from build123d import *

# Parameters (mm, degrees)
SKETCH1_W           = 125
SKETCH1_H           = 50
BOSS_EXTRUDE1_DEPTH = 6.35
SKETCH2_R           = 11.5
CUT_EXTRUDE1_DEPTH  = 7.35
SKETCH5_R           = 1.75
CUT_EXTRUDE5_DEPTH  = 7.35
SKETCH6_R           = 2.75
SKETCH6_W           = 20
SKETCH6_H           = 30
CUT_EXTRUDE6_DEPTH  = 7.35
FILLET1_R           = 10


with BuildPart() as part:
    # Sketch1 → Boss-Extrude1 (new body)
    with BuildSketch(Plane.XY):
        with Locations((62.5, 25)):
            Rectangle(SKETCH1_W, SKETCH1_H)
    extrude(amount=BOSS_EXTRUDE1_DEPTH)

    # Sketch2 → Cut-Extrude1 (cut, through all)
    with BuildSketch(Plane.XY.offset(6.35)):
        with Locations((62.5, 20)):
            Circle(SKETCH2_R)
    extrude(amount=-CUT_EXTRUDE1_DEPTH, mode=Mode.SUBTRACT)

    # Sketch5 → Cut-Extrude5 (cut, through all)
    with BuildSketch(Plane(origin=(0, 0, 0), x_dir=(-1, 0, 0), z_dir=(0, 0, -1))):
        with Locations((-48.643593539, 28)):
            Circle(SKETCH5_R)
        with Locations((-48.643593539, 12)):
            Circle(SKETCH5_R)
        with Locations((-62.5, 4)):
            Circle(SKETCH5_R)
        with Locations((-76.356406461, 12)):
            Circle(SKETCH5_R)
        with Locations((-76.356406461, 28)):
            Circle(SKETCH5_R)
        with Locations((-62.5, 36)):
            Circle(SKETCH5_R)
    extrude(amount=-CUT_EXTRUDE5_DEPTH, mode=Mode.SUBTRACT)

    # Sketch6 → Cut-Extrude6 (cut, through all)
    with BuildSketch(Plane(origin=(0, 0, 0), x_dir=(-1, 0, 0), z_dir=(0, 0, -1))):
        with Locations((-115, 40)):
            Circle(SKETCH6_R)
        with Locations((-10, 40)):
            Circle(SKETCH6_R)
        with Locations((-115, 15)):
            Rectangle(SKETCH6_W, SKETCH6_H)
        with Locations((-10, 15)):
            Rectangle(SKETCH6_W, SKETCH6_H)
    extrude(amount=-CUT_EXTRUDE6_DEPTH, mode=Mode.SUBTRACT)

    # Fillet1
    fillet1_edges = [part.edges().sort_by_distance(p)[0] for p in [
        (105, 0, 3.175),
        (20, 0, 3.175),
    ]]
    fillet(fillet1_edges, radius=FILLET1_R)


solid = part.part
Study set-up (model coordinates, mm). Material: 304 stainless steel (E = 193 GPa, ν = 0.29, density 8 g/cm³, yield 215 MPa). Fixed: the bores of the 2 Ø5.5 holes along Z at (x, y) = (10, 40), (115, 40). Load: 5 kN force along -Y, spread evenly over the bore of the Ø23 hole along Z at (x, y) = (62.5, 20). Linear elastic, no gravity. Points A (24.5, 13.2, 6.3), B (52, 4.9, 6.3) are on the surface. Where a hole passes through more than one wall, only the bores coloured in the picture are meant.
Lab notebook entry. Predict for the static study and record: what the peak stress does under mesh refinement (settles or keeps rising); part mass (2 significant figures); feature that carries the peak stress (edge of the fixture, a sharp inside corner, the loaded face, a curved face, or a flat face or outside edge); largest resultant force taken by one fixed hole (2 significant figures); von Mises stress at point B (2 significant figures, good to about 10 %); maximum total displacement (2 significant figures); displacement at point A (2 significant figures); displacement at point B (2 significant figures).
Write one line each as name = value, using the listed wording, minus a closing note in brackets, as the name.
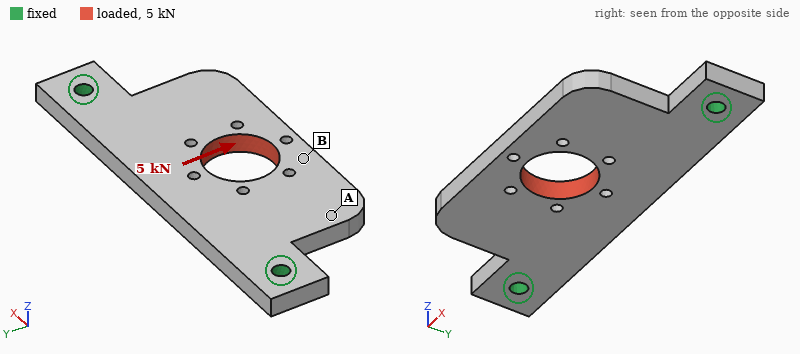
what the peak stress does under mesh refinement = keeps rising
part mass = 230 g
feature that carries the peak stress = edge of the fixture
largest resultant force taken by one fixed hole = 2.9 kN
von Mises stress at point B = 34 MPa
maximum total displacement = 19 µm
displacement at point A = 11 µm
displacement at point B = 16 µm
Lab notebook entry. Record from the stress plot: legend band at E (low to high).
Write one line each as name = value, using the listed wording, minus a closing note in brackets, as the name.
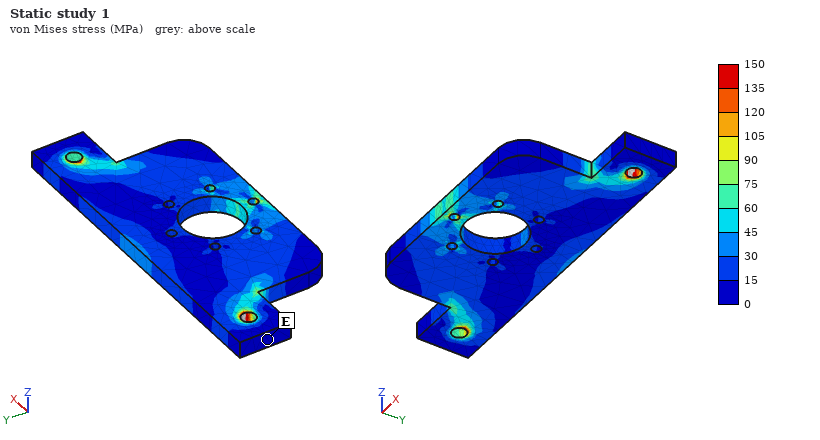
legend band at E = 0 to 15 MPa
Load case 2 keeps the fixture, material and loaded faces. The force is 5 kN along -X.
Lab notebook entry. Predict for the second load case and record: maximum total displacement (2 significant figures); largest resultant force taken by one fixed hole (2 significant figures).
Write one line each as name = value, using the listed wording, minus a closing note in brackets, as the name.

maximum total displacement = 9.2 µm
largest resultant force taken by one fixed hole = 2.7 kN
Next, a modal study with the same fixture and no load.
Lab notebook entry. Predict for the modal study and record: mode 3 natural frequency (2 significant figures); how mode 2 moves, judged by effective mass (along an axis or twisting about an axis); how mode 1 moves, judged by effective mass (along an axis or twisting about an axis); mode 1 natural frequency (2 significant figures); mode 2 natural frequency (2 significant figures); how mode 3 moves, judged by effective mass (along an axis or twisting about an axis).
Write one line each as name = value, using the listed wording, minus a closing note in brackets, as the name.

mode 3 natural frequency = 3700 Hz
how mode 2 moves, judged by effective mass = along Z
how mode 1 moves, judged by effective mass = along Z
mode 1 natural frequency = 1500 Hz
mode 2 natural frequency = 3200 Hz
how mode 3 moves, judged by effective mass = twisting about Y
